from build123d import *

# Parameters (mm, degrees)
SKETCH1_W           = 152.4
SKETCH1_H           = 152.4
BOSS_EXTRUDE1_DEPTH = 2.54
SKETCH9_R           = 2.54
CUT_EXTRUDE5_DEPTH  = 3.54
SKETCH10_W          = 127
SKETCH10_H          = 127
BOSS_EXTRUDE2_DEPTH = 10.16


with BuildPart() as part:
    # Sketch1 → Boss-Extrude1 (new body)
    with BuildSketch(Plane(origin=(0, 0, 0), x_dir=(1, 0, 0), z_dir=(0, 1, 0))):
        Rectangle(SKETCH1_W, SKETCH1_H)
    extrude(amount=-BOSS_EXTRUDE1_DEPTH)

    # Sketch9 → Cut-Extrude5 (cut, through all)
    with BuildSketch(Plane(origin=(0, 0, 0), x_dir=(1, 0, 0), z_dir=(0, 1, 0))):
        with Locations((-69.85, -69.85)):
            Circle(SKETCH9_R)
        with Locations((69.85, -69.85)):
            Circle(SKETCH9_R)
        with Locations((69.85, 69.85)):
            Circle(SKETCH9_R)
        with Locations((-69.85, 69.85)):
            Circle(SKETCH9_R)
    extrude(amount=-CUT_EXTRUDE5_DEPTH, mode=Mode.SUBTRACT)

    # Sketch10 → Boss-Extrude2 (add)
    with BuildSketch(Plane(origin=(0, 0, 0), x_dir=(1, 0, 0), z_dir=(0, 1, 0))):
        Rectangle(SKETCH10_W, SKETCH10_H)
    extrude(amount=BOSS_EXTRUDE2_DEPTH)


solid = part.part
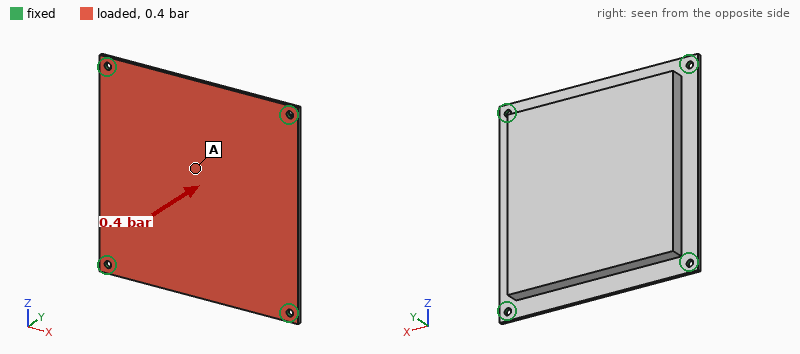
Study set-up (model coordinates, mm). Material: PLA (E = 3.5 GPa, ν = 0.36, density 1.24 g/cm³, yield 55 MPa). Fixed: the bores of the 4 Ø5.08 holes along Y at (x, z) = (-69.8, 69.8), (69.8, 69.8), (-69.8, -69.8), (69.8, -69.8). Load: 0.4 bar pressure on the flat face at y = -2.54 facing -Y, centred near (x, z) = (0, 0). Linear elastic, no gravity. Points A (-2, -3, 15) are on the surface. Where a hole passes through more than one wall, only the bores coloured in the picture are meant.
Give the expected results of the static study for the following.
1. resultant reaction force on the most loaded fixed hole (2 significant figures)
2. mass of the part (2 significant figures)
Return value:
430 N
280 g
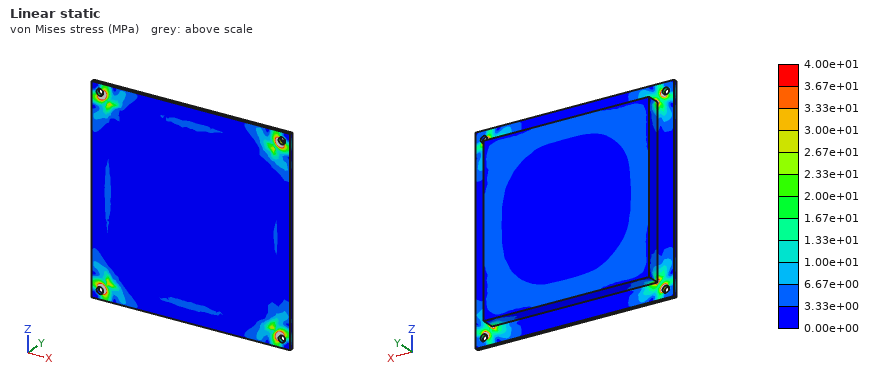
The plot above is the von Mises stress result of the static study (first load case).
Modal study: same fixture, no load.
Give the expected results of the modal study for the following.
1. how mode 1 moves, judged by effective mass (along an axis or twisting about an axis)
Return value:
along Y
